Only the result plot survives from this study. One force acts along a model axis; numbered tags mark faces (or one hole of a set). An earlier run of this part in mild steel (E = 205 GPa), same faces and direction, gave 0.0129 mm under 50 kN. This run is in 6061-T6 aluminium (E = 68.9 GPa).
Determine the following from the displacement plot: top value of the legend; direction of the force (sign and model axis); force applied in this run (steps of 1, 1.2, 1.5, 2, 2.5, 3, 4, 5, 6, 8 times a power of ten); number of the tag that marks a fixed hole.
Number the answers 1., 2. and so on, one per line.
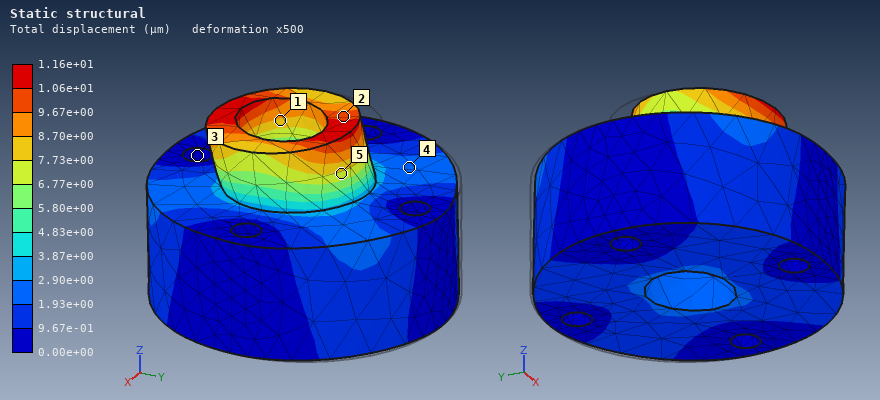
1. 1.16e+01 µm
2. -Y
3. 15 kN
4. 3
